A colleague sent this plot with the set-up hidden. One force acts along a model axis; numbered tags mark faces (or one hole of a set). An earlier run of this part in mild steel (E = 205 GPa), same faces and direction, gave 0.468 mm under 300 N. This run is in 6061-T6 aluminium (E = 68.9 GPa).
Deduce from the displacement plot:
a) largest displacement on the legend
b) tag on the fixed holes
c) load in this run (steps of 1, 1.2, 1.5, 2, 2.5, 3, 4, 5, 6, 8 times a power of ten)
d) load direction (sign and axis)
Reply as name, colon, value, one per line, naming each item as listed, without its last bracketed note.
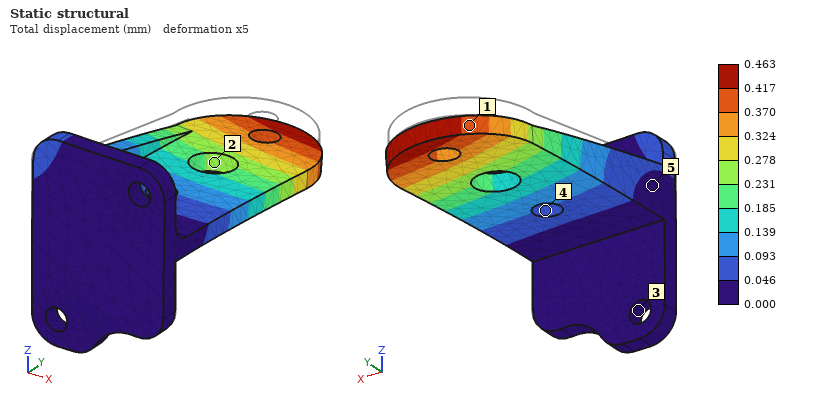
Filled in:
largest displacement on the legend: 0.463 mm
tag on the fixed holes: 3
load in this run: 100 N
load direction: -Z
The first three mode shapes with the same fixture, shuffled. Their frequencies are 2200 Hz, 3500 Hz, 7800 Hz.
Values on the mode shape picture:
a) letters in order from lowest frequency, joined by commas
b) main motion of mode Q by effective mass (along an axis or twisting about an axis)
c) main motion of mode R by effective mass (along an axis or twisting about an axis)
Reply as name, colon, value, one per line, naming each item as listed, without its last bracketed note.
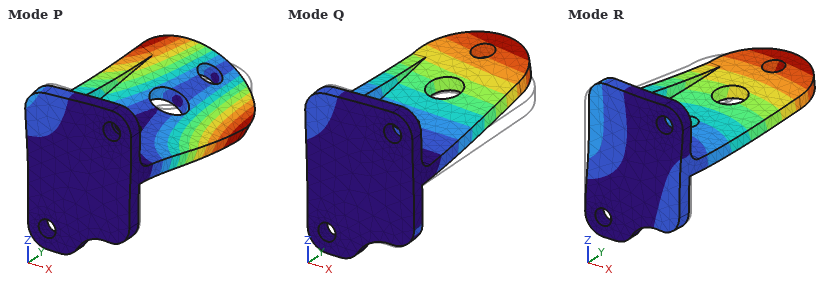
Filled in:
letters in order from lowest frequency, joined by commas: Q, R, P
main motion of mode Q by effective mass: along Z
main motion of mode R by effective mass: along X
